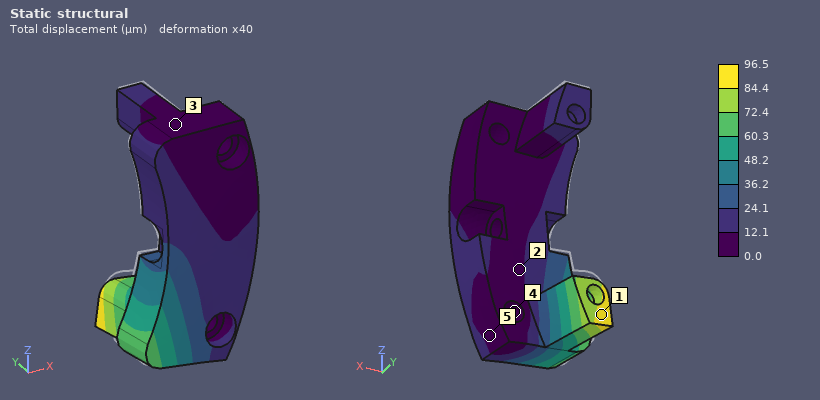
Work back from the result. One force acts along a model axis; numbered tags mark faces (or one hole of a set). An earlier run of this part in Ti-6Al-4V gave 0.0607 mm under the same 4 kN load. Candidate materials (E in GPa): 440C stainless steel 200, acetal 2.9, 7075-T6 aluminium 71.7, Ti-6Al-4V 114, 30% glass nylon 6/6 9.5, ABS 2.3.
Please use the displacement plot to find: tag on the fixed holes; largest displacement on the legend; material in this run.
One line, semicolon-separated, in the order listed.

4; 96.5 µm; 7075-T6 aluminium
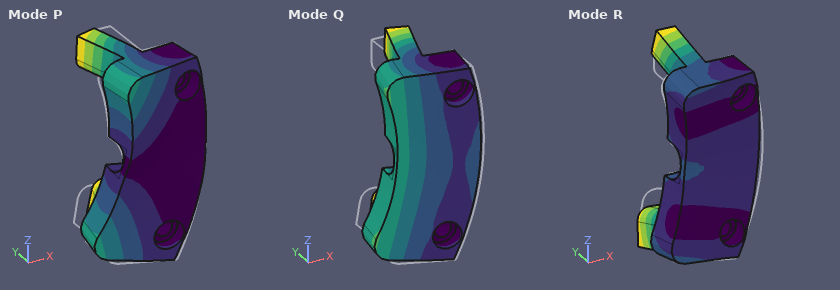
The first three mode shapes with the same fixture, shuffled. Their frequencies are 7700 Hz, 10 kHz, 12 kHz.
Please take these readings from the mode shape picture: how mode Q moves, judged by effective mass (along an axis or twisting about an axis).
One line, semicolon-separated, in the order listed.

along Y
